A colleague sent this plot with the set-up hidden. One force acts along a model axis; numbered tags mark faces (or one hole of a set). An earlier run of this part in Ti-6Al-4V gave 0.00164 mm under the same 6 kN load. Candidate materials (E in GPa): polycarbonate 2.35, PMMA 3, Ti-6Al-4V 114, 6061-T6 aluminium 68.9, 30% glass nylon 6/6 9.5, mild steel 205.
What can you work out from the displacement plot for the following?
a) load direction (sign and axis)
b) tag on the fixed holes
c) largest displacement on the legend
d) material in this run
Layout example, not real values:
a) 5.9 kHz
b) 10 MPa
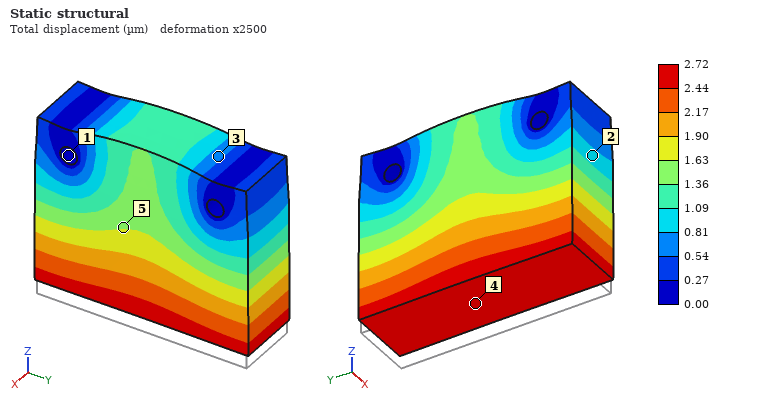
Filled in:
a) +Z
b) 1
c) 2.72 µm
d) 6061-T6 aluminium
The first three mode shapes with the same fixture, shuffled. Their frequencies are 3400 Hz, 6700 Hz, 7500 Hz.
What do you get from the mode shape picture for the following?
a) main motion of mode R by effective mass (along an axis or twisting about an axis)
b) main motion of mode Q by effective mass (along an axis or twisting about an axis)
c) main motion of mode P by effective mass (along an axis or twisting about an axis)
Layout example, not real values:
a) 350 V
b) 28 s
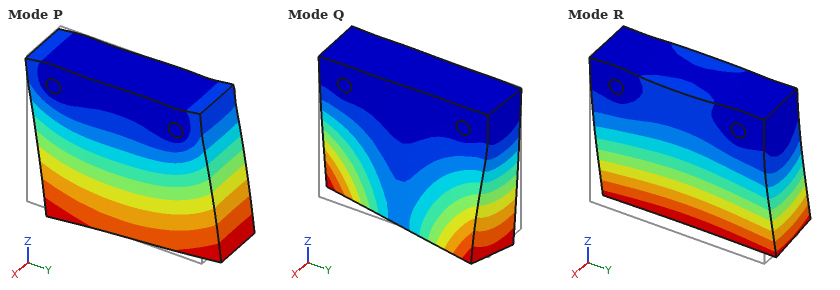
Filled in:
a) along X
b) twisting about Z
c) along Y
